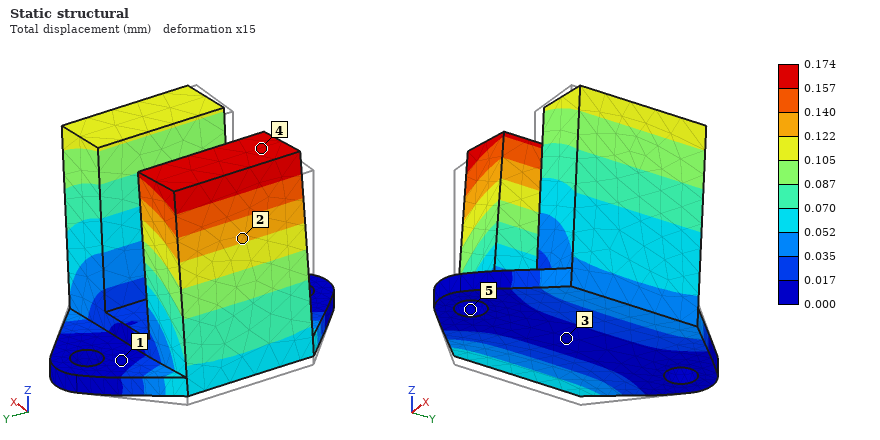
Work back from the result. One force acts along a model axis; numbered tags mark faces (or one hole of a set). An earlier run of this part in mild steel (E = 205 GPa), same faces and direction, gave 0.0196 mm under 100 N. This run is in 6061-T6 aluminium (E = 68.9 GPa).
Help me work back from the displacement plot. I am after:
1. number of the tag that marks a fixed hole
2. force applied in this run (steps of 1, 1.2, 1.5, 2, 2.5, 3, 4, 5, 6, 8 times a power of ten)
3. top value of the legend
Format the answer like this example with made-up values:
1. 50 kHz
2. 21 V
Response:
1. 5
2. 300 N
3. 0.174 mm
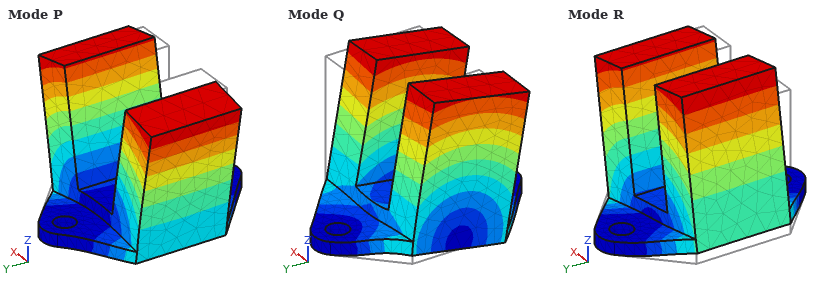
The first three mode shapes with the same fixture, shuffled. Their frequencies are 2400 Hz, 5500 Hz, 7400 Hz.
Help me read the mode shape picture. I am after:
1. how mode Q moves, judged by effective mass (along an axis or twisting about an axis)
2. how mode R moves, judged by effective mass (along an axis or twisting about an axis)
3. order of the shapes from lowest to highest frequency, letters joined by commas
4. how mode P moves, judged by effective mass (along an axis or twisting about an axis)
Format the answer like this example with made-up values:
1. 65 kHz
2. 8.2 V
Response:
1. along Y
2. along X
3. R, P, Q
4. along Z
